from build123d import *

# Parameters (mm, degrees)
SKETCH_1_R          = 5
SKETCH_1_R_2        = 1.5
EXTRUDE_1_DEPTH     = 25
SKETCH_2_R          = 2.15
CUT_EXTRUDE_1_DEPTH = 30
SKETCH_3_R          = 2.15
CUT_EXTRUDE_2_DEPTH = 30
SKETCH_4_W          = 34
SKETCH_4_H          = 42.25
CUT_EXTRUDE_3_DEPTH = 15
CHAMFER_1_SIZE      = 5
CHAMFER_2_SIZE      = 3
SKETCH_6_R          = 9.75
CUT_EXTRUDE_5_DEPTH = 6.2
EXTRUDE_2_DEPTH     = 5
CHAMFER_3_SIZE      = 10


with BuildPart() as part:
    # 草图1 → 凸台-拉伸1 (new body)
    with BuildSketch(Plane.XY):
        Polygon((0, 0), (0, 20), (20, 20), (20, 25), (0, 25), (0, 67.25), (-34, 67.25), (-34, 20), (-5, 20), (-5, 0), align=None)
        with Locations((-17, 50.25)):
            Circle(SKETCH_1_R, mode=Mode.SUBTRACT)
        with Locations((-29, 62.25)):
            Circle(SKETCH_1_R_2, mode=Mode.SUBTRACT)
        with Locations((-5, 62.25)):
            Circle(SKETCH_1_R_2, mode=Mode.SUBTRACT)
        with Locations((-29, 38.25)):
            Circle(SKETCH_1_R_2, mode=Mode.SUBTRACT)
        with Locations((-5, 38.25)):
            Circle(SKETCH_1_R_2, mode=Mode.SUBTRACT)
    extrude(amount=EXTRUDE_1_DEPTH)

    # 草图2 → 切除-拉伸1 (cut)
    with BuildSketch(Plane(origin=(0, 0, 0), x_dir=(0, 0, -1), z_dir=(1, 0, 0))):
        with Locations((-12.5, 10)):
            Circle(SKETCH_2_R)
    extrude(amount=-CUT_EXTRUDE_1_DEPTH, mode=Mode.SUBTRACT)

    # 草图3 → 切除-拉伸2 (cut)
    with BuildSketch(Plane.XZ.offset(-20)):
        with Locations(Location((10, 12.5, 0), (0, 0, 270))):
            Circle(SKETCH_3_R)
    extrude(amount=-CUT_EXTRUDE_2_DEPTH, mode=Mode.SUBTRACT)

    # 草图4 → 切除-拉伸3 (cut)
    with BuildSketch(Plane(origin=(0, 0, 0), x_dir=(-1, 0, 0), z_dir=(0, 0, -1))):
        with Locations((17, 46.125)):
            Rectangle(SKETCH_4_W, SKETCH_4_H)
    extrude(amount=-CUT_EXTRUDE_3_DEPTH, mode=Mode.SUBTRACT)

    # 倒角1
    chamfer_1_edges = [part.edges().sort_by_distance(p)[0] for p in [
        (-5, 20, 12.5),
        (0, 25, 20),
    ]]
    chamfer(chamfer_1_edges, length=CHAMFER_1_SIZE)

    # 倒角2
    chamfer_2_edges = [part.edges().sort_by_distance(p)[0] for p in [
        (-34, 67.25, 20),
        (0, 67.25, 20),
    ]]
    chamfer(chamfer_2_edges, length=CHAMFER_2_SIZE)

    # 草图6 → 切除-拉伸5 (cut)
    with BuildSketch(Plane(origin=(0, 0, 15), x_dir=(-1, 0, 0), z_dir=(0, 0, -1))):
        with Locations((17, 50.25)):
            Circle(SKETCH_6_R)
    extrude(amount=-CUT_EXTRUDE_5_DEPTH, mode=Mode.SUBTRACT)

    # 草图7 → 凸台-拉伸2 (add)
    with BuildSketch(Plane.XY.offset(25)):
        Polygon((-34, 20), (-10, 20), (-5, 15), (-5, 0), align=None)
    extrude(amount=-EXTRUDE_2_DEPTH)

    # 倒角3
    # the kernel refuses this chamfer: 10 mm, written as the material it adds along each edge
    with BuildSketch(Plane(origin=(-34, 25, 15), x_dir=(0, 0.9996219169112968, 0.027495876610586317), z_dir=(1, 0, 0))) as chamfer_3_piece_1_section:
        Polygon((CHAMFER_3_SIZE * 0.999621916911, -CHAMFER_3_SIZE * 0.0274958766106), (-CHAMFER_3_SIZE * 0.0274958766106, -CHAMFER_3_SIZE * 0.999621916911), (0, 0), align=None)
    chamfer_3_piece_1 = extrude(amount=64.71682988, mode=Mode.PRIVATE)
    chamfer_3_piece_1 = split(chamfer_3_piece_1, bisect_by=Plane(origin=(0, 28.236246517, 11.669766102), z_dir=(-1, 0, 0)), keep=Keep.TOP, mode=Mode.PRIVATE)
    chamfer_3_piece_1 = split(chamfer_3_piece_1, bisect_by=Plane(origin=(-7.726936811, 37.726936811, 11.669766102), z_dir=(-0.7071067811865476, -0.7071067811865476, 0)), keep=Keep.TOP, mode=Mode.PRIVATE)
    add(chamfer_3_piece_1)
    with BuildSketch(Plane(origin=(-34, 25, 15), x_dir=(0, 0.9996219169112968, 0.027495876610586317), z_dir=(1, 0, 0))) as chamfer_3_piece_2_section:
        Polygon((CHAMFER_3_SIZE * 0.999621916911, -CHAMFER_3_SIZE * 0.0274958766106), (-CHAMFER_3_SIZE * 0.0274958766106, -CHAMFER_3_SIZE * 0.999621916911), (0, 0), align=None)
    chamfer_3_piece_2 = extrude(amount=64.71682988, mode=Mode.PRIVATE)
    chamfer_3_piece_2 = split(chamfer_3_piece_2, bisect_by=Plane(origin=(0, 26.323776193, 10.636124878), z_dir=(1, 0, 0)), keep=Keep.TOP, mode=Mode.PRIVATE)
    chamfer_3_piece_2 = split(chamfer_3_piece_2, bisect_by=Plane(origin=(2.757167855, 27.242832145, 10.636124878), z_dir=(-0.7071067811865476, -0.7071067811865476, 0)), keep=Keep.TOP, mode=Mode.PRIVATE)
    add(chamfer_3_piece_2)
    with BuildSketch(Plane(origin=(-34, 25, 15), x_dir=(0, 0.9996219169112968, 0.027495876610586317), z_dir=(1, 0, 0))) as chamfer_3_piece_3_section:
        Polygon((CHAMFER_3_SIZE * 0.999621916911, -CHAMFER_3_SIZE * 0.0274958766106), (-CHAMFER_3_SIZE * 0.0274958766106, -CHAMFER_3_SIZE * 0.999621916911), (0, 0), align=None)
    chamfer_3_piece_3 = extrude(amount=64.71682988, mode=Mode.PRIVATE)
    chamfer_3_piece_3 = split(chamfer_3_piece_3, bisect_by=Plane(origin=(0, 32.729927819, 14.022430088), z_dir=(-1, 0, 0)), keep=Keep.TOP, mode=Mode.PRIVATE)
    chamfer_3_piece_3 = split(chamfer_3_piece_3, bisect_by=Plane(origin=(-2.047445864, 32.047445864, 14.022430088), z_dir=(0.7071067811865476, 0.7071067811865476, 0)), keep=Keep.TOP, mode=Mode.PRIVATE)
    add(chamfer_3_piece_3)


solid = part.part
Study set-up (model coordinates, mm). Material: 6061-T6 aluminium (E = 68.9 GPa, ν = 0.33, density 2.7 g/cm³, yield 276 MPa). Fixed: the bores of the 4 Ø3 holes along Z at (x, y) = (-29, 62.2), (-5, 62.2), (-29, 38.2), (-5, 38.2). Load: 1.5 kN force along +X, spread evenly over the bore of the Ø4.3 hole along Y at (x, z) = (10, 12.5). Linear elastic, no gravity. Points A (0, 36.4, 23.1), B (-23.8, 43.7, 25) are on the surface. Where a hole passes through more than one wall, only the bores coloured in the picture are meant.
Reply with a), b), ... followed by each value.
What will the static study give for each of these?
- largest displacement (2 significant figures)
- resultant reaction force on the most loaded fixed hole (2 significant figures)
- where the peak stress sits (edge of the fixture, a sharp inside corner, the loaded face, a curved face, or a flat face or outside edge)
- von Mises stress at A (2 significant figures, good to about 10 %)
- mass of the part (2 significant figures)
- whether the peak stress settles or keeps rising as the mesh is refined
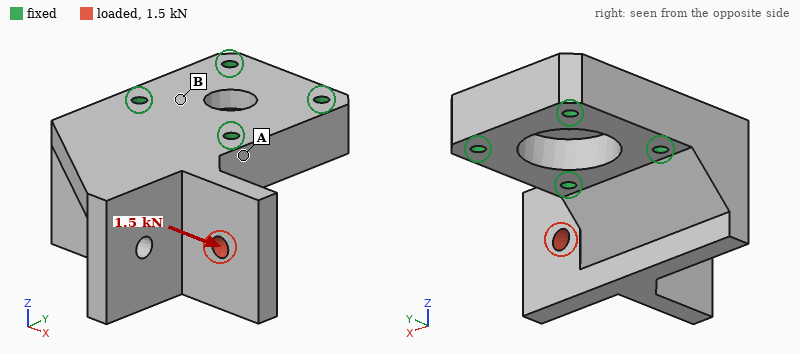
a) 15 µm
b) 1.2 kN
c) edge of the fixture
d) 11 MPa
e) 66 g
f) keeps rising
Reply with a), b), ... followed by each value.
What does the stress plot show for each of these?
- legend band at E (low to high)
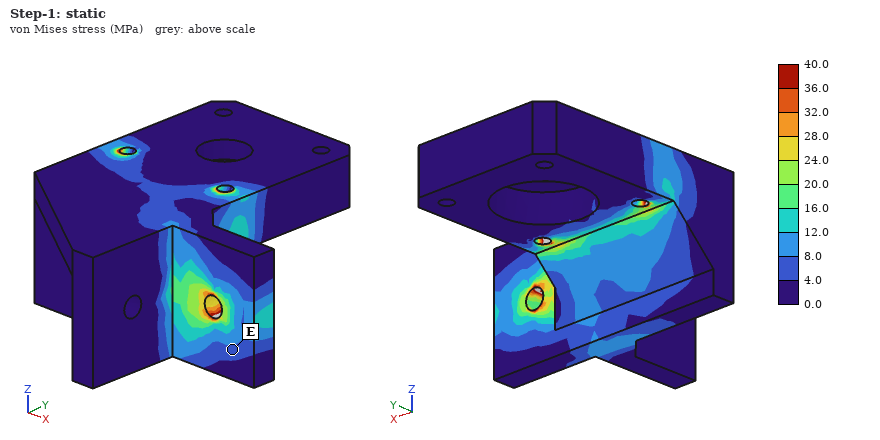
a) 4.0 to 8.0 MPa
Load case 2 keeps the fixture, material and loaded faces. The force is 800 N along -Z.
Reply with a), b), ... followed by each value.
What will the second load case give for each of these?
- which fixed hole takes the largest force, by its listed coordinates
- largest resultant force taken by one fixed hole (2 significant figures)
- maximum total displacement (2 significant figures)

a) (-5, 38.2)
b) 1.2 kN
c) 42 µm
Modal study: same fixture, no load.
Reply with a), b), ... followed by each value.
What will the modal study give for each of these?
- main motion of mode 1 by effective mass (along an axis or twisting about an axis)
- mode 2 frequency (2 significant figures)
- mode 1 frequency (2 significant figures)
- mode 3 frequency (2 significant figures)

a) along Z
b) 9200 Hz
c) 5200 Hz
d) 11 kHz
